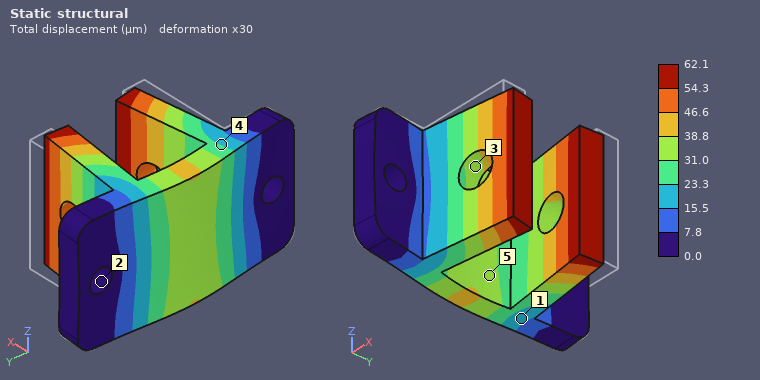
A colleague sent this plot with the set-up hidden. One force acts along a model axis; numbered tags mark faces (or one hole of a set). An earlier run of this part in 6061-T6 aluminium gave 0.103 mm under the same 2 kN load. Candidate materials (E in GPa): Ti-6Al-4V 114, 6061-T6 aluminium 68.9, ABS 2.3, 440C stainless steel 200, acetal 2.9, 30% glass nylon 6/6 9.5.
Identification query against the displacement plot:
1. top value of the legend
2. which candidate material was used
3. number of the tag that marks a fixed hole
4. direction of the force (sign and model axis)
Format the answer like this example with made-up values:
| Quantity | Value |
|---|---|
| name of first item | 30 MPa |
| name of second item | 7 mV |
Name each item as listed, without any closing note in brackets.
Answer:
| Quantity | Value |
|---|---|
| top value of the legend | 62.1 µm |
| which candidate material was used | Ti-6Al-4V |
| number of the tag that marks a fixed hole | 2 |
| direction of the force | -X |
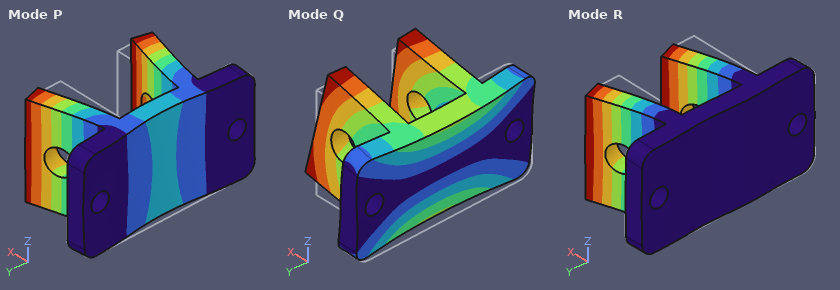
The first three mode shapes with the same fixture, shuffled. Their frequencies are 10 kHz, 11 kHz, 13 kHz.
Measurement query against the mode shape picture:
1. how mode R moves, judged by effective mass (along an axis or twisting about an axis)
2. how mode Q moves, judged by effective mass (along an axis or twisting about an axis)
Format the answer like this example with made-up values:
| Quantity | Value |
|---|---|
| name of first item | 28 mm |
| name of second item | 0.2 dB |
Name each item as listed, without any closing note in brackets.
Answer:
| Quantity | Value |
|---|---|
| how mode R moves, judged by effective mass | along Y |
| how mode Q moves, judged by effective mass | along Z |
